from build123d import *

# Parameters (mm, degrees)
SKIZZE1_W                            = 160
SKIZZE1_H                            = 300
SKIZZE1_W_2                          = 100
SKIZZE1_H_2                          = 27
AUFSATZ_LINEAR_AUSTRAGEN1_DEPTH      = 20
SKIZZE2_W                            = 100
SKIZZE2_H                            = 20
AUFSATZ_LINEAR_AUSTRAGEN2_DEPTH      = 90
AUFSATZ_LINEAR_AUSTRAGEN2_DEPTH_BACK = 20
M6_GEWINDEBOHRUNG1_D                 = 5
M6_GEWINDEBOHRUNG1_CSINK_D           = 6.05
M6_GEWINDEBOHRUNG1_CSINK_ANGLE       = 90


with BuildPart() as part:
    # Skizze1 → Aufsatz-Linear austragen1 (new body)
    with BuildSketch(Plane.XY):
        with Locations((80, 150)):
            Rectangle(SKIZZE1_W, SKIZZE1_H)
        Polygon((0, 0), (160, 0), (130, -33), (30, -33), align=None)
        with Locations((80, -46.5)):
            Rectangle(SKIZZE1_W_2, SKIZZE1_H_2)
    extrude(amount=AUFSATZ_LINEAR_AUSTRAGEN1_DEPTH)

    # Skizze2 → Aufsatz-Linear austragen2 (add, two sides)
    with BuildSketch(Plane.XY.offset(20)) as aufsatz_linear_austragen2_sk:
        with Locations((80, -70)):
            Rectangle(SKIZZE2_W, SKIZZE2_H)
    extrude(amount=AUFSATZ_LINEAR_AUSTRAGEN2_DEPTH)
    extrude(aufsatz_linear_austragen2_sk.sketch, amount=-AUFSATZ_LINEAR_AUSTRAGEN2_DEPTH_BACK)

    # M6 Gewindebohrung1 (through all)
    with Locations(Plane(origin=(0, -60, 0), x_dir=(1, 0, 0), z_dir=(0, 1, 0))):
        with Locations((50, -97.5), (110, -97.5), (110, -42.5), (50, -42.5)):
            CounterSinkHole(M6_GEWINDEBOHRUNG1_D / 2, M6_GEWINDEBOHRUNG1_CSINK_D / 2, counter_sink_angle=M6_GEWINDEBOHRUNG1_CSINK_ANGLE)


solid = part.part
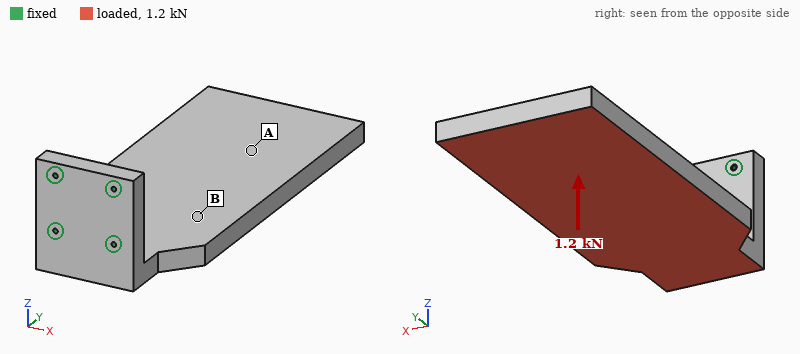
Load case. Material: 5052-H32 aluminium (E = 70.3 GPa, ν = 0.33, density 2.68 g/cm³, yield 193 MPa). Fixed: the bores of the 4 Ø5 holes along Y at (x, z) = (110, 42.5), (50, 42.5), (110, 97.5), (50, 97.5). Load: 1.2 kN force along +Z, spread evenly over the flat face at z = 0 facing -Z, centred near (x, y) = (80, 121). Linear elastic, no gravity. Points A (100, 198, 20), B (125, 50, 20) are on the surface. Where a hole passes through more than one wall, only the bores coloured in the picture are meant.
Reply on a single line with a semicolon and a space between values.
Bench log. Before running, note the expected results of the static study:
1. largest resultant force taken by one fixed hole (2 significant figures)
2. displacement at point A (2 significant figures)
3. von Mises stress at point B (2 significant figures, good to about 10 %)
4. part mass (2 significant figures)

1.2 kN; 1.3 mm; 9.6 MPa; 3.5 kg
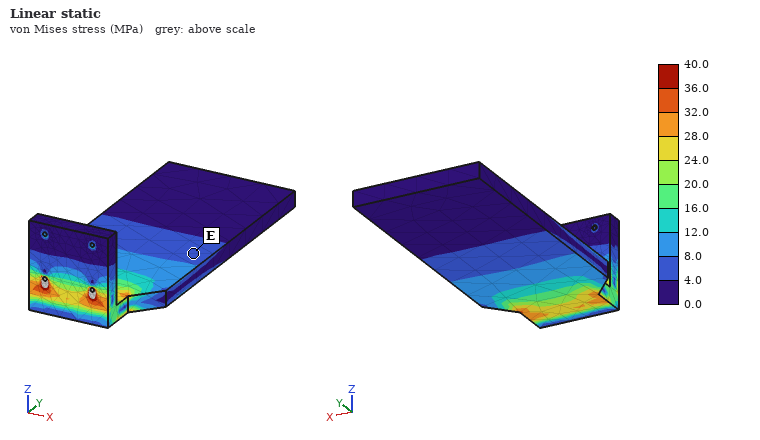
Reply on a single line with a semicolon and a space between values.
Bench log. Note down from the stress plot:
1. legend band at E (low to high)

4.0 to 8.0 MPa
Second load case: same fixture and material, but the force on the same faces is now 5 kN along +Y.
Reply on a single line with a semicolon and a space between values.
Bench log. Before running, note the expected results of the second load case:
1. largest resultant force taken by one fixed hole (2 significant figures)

3.4 kN
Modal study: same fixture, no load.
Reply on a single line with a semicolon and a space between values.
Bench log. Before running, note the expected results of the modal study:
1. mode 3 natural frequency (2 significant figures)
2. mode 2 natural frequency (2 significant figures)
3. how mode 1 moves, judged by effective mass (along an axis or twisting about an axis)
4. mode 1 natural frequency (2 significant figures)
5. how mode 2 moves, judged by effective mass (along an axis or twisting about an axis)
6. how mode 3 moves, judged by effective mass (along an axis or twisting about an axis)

500 Hz; 260 Hz; along Z; 90 Hz; along X; twisting about Y
